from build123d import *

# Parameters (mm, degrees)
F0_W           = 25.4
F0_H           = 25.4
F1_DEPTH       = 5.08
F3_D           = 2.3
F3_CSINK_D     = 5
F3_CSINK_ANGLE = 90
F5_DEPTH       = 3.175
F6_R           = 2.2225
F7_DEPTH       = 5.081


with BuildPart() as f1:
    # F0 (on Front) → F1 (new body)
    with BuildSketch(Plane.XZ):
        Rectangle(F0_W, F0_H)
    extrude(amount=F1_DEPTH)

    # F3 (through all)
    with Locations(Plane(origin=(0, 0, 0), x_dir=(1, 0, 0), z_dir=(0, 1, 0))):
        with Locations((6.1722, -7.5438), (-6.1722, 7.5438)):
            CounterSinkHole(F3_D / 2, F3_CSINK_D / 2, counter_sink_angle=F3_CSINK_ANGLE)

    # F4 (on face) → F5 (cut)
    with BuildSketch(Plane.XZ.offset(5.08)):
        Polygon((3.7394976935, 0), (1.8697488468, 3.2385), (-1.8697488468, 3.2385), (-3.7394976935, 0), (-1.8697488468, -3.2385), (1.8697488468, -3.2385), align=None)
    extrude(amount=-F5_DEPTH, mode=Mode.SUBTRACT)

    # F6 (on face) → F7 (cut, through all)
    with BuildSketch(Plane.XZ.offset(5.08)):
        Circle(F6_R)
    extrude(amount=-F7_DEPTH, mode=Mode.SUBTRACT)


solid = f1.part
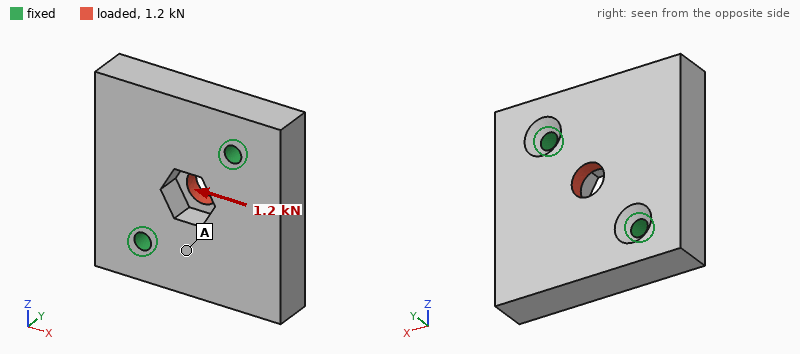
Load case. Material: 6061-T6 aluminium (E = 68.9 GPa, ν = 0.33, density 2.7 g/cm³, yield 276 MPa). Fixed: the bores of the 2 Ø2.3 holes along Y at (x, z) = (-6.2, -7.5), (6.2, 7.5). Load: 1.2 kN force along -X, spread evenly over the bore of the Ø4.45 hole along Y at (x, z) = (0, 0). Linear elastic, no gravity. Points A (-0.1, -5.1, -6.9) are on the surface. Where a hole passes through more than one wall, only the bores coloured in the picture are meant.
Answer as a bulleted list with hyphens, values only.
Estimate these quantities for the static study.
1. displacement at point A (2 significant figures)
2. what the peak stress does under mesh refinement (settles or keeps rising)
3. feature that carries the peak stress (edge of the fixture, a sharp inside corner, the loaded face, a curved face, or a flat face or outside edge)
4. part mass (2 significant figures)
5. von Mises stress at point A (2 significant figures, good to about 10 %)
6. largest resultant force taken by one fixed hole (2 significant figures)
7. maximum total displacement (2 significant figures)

- 2.1 µm
- keeps rising
- edge of the fixture
- 8.3 g
- 10.0 MPa
- 600 N
- 11 µm
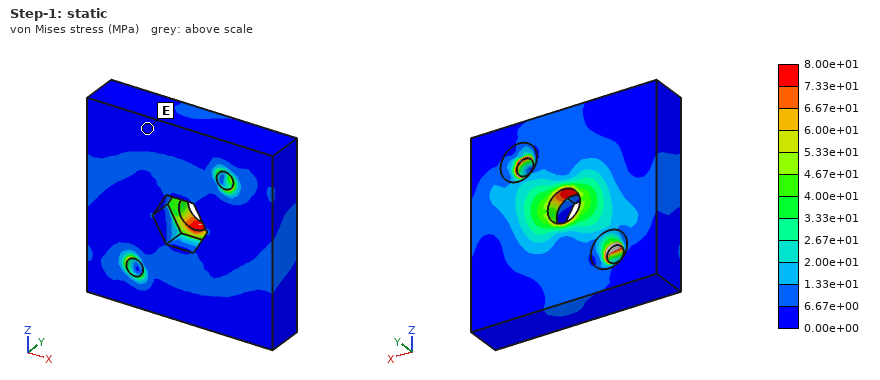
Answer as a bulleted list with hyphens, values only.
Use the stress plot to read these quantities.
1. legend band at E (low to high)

- 0.00e+00 to 6.67e+00 MPa
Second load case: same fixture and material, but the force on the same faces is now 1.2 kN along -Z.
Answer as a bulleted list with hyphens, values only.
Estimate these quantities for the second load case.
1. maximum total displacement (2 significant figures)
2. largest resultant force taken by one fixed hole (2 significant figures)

- 9.7 µm
- 610 N
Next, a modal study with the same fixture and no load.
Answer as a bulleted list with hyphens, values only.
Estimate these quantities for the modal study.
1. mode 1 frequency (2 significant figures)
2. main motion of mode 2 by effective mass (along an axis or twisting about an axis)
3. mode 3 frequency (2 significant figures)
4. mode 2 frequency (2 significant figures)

- 13 kHz
- along Y
- 40 kHz
- 18 kHz
